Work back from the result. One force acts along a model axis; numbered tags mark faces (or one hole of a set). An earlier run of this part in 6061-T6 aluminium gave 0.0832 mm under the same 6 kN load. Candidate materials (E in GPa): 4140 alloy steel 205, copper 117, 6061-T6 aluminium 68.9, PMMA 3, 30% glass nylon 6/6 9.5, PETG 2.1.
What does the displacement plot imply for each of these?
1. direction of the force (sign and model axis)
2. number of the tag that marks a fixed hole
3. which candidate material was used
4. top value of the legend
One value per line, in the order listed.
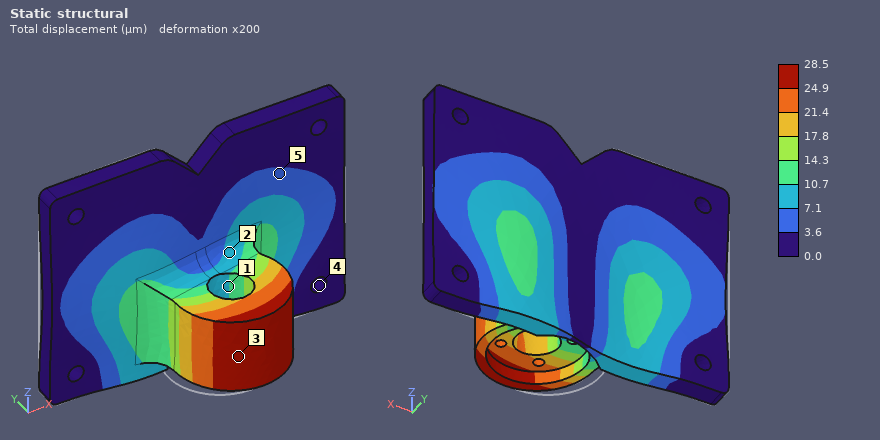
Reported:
+X
4
4140 alloy steel
28.5 µm
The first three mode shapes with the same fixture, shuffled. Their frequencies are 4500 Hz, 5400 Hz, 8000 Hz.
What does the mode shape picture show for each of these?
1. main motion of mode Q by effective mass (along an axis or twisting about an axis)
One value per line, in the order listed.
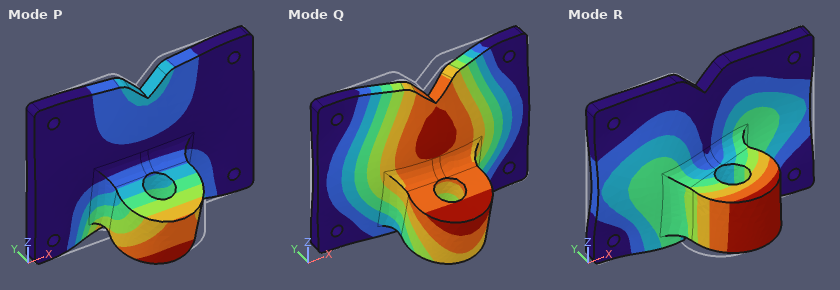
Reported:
along Y
